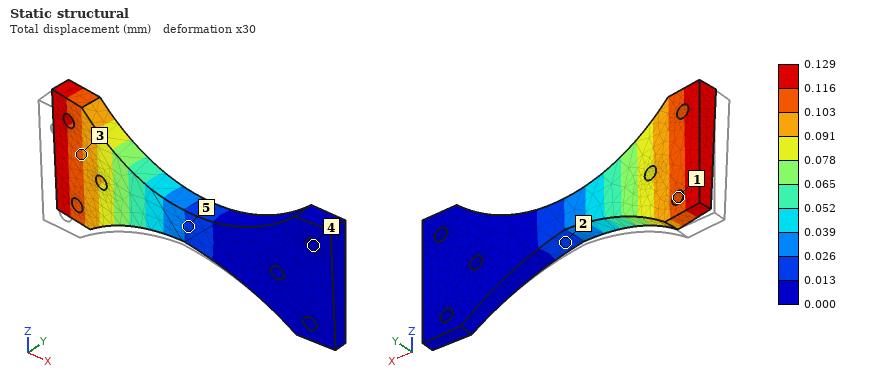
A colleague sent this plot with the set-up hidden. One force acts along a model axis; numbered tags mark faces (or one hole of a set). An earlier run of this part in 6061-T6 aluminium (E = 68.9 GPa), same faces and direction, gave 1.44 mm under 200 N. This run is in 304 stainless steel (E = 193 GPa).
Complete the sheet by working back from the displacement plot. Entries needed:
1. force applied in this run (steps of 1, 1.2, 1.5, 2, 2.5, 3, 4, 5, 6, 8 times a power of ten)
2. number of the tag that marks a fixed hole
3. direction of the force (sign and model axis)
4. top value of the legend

50 N
4
+Y
0.129 mm
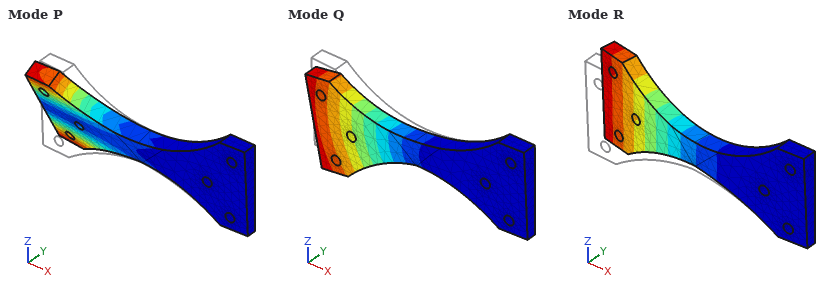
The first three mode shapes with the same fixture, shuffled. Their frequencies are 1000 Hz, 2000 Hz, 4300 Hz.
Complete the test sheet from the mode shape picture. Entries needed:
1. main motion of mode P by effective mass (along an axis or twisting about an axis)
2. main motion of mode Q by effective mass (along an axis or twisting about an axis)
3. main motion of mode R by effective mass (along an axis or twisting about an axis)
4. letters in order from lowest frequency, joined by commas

twisting about X
along Z
along Y
R, Q, P
